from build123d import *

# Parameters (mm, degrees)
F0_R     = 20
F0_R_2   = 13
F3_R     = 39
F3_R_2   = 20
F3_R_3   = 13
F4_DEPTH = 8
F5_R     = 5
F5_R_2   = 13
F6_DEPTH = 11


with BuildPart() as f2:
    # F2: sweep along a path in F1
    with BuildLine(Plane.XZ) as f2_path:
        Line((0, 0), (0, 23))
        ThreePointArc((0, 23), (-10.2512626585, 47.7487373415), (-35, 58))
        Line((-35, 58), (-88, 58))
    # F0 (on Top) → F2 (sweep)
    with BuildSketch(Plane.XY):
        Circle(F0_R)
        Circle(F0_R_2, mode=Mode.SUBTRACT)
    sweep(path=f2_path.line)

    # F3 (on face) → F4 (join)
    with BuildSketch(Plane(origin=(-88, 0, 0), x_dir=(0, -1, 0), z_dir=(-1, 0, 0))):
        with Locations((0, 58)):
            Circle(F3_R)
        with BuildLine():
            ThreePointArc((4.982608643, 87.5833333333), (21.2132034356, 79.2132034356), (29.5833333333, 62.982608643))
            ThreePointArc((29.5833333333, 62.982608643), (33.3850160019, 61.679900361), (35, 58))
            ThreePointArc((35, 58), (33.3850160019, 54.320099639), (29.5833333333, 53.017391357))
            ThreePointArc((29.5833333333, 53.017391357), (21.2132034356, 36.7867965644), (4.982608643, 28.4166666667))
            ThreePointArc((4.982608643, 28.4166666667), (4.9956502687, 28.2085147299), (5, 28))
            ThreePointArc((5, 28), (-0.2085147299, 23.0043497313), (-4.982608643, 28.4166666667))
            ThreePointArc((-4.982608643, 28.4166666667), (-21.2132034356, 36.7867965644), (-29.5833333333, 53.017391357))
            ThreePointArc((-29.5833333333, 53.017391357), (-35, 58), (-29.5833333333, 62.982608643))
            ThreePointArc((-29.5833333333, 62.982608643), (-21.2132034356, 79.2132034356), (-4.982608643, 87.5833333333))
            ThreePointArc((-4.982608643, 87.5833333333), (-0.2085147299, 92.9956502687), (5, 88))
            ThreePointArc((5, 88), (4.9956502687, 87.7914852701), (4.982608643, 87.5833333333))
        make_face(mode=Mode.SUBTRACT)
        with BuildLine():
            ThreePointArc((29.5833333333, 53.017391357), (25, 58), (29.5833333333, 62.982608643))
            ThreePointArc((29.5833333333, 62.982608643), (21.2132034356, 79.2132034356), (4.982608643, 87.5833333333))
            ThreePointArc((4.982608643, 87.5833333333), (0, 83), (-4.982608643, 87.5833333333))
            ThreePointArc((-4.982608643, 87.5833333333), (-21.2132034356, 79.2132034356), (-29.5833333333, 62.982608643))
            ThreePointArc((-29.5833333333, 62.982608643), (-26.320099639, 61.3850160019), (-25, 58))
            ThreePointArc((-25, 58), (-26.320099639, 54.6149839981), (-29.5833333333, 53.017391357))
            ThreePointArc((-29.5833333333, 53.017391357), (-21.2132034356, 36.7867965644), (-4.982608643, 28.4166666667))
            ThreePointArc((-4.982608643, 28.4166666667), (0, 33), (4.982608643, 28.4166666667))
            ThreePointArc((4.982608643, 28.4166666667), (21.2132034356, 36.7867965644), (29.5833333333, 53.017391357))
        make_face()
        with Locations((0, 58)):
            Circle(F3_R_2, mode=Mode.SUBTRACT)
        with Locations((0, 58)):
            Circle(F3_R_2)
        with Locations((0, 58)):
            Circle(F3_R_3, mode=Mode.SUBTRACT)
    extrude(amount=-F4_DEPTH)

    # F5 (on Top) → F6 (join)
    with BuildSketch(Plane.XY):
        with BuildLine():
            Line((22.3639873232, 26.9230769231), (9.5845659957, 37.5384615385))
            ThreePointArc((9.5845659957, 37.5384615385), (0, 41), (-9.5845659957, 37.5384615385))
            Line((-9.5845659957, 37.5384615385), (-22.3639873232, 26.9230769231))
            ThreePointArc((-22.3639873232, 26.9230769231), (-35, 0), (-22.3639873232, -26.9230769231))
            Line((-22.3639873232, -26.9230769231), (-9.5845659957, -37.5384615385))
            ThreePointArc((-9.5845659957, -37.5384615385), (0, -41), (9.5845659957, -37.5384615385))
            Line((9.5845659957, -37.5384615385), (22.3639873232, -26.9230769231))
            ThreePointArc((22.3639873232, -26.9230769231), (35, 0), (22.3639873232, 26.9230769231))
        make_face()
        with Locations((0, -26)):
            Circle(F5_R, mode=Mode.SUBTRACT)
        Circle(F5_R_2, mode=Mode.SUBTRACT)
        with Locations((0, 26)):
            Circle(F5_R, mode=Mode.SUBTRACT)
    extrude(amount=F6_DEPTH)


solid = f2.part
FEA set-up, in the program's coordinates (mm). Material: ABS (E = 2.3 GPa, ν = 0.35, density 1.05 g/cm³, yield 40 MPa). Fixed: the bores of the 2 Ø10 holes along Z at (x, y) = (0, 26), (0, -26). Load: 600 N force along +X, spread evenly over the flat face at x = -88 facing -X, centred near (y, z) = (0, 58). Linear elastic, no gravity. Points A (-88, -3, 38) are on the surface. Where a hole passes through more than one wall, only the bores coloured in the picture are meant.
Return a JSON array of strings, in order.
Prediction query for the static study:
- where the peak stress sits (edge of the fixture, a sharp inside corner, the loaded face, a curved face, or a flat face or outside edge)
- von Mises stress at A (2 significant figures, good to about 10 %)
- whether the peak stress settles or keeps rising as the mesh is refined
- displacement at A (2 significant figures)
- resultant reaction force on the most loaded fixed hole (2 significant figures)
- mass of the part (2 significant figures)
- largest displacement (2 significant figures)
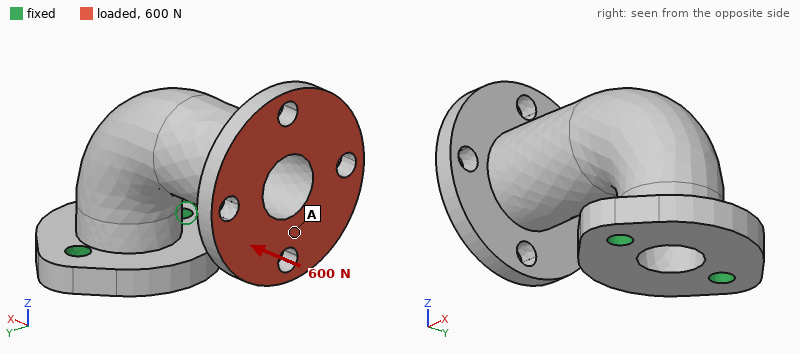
["edge of the fixture", "2.5 MPa", "keeps rising", "1.4 mm", "300 N", "160 g", "2.0 mm"]
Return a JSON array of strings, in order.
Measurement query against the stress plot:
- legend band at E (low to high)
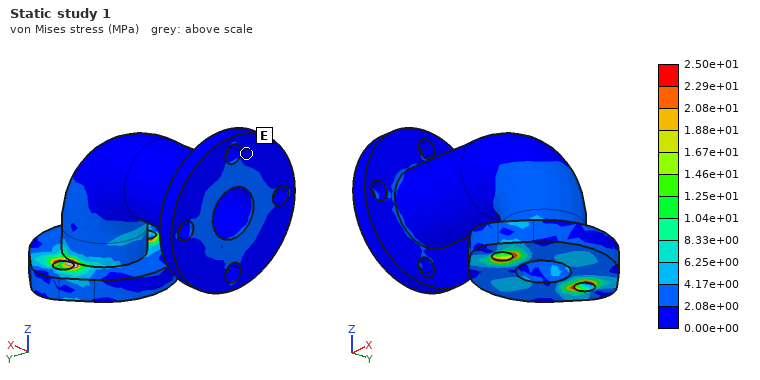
["0.00e+00 to 2.08e+00 MPa"]
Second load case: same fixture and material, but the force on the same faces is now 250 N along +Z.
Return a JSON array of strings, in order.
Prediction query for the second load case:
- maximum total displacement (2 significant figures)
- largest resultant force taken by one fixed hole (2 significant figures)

["1.9 mm", "160 N"]
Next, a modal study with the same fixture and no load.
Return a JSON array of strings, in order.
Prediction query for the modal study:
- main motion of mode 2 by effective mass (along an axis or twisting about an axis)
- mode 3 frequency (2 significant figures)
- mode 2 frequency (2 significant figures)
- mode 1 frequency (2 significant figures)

["along Y", "960 Hz", "390 Hz", "260 Hz"]
